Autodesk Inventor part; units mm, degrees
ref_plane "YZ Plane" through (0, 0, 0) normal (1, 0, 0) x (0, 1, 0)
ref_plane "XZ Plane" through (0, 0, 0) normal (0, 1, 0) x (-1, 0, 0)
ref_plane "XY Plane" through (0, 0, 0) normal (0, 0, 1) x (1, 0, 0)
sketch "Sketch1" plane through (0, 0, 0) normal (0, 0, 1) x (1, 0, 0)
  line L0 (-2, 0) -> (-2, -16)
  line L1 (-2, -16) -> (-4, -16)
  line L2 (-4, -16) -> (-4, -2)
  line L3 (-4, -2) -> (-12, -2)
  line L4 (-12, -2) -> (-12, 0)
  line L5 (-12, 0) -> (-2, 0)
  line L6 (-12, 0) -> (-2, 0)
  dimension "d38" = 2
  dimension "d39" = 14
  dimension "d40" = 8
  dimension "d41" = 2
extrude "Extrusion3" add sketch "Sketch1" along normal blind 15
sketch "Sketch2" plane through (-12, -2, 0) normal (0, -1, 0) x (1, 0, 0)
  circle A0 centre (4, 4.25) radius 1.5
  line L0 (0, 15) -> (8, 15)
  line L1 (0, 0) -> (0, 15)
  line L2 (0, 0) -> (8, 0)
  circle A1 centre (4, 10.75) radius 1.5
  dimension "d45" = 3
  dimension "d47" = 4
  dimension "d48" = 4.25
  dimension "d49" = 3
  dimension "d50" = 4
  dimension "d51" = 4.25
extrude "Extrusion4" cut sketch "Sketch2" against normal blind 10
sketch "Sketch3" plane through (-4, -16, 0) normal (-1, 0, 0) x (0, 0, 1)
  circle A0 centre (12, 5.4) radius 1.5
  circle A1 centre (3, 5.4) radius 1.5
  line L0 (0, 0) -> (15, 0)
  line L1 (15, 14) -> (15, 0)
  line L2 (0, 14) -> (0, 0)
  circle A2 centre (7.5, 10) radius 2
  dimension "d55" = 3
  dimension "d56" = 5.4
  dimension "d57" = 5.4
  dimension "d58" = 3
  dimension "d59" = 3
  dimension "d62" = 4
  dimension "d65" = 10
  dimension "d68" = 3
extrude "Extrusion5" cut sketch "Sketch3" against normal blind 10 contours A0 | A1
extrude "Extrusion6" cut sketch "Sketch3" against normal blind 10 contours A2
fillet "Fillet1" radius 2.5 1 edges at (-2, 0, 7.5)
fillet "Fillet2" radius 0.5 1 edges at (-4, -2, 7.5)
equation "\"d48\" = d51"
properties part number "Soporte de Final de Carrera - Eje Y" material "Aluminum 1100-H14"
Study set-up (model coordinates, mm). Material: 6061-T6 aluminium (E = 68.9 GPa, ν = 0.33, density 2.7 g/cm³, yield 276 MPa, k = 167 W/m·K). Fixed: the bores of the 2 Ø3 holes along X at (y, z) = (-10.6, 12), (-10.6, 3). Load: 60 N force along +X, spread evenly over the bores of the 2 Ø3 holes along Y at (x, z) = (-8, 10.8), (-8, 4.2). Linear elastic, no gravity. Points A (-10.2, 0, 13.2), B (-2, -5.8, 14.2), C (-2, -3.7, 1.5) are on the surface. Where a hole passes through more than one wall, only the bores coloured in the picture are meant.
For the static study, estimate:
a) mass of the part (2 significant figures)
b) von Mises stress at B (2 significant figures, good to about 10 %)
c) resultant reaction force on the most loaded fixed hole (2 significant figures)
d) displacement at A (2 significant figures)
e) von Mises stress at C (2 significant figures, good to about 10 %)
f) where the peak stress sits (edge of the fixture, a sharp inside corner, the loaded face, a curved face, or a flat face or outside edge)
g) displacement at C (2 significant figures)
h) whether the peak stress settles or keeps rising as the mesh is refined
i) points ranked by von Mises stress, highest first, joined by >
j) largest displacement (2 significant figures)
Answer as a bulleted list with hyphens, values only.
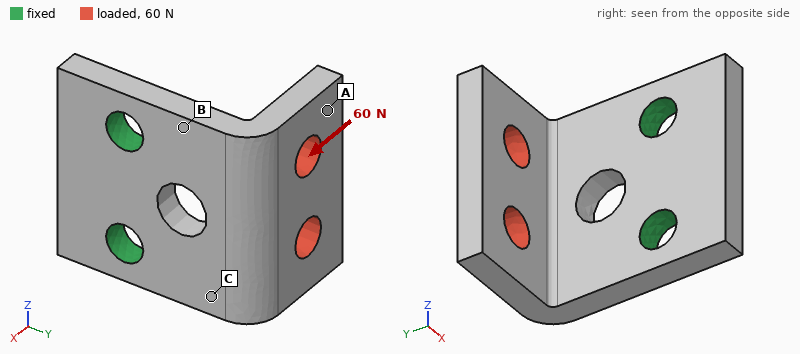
- 1.7 g
- 36 MPa
- 30 N
- 39 µm
- 20 MPa
- edge of the fixture
- 13 µm
- keeps rising
- B > C > A
- 44 µm
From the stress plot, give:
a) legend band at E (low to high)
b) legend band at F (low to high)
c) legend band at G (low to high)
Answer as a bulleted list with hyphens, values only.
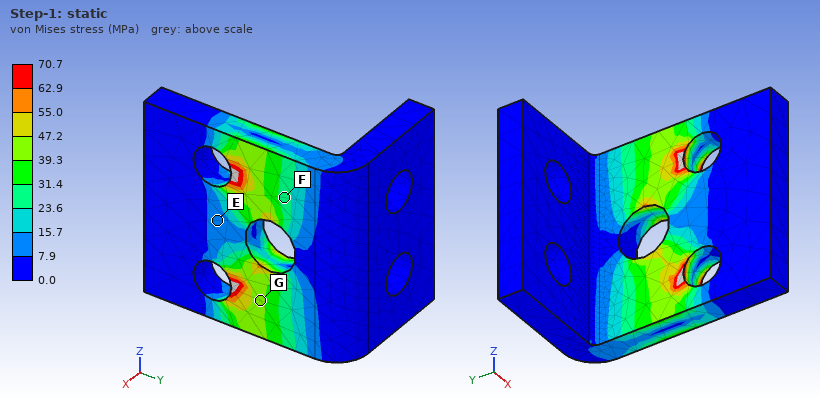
- 7.9 to 15.7 MPa
- 23.6 to 31.4 MPa
- 39.3 to 47.2 MPa
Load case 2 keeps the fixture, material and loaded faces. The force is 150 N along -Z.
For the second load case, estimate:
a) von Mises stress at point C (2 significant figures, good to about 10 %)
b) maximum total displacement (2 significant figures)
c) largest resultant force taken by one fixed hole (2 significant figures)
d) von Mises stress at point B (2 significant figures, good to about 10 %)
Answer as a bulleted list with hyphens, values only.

- 32 MPa
- 46 µm
- 150 N
- 36 MPa
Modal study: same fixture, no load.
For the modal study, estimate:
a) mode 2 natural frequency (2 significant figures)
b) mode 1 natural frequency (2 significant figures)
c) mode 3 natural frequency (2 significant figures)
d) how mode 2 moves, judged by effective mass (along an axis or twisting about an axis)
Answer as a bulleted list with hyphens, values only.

- 12 kHz
- 6900 Hz
- 20 kHz
- along Z
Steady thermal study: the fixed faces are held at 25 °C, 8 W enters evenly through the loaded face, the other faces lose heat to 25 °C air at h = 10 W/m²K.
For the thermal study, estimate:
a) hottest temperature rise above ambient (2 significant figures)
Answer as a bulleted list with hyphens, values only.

- 26 K
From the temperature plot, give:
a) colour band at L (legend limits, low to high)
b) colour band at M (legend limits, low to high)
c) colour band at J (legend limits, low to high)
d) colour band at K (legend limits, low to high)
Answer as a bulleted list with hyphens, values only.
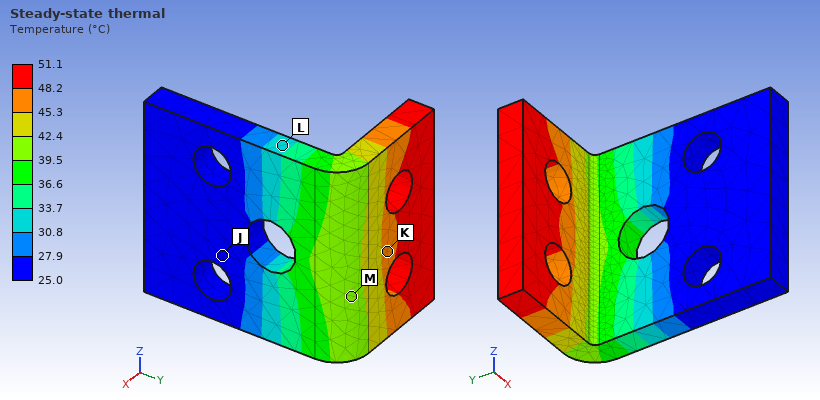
- 30.8 to 33.7 °C
- 39.5 to 42.4 °C
- 25.0 to 27.9 °C
- 45.3 to 48.2 °C
